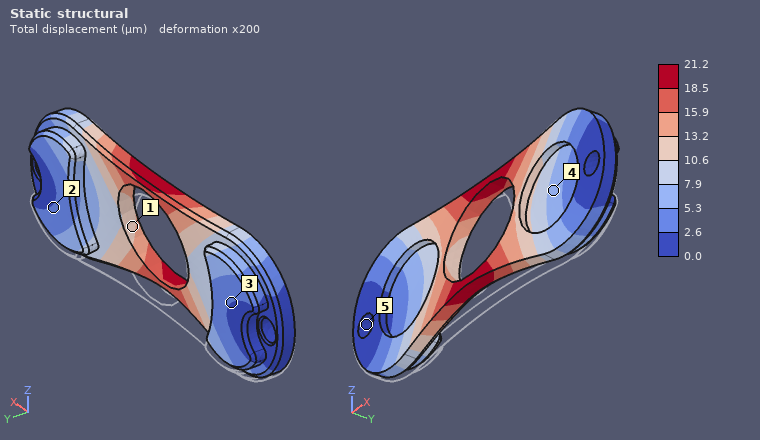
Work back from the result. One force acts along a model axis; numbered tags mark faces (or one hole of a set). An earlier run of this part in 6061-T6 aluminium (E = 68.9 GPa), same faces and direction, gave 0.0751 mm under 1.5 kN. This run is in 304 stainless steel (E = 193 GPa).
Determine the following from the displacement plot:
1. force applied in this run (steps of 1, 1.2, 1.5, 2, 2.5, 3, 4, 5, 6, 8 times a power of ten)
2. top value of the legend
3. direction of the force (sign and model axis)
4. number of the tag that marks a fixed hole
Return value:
1.2 kN
21.2 µm
+Z
5
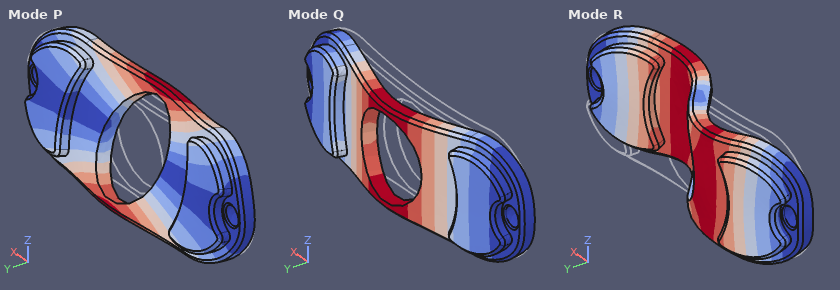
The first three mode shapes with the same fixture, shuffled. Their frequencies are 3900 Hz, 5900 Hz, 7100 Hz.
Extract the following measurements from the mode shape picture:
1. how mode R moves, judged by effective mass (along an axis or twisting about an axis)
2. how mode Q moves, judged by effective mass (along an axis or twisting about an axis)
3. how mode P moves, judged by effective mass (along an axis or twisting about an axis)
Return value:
twisting about Z
along Y
twisting about X
